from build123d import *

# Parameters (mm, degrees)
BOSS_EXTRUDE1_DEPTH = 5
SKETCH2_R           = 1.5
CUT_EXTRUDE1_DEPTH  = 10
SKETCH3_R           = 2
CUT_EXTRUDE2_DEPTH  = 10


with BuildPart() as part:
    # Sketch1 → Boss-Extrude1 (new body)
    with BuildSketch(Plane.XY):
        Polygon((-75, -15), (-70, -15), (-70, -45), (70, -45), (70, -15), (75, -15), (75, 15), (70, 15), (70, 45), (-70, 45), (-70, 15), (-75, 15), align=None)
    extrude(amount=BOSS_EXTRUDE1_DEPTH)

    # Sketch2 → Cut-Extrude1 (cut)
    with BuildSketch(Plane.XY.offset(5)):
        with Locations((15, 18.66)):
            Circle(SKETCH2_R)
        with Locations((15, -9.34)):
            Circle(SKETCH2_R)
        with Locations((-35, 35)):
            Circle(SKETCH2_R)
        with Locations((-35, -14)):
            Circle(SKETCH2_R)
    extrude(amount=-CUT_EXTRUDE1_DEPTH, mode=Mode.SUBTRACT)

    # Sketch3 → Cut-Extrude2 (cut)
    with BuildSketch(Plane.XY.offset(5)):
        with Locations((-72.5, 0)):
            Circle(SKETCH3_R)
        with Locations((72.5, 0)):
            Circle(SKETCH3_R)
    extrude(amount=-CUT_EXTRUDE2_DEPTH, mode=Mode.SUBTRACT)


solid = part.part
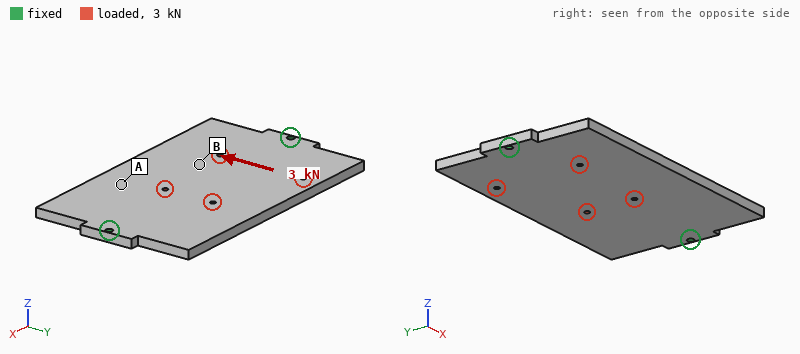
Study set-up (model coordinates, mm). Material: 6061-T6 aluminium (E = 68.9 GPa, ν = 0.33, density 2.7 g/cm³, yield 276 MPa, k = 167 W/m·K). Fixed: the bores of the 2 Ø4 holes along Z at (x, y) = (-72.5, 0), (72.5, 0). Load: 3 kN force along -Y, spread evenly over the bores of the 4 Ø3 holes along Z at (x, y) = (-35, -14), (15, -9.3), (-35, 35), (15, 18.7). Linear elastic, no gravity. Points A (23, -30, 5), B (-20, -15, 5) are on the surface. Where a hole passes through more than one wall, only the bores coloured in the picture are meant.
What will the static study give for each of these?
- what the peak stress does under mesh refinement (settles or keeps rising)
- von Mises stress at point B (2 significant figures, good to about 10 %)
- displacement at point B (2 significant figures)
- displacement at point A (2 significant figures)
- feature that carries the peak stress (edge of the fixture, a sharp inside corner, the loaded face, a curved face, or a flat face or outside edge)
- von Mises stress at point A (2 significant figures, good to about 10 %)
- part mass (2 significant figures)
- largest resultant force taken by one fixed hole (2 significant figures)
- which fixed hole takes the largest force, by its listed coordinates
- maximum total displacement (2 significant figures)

keeps rising
3.5 MPa
17 µm
15 µm
edge of the fixture
7.5 MPa
170 g
1.7 kN
(-72.5, 0)
18 µm
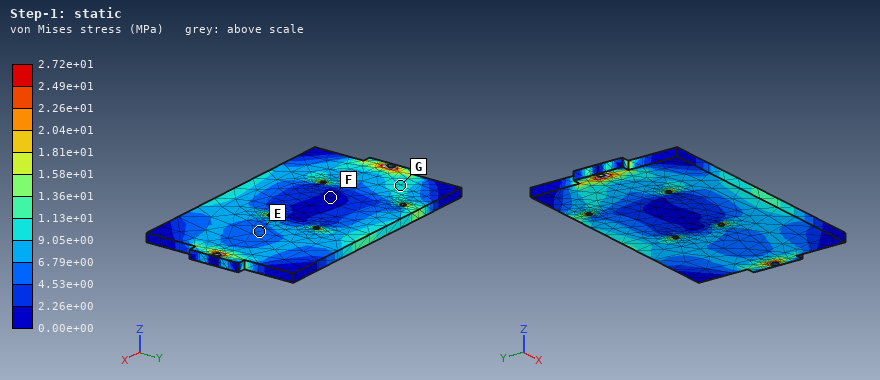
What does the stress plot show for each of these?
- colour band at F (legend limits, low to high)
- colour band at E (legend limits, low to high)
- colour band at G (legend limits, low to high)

0.00e+00 to 2.26e+00 MPa
4.53e+00 to 6.79e+00 MPa
9.05e+00 to 1.13e+01 MPa
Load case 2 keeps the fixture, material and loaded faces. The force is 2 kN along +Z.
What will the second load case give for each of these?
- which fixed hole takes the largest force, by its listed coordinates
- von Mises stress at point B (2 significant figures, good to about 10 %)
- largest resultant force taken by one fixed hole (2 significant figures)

(-72.5, 0)
51 MPa
1.2 kN
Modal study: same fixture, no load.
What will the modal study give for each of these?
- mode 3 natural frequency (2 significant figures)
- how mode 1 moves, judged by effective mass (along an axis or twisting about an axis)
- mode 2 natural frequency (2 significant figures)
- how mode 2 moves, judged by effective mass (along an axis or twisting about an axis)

1800 Hz
twisting about X
820 Hz
along Z
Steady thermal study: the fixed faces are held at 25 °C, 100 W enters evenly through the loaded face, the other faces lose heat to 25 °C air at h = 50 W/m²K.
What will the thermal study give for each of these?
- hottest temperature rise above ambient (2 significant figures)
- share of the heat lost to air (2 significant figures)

51 K
43 %
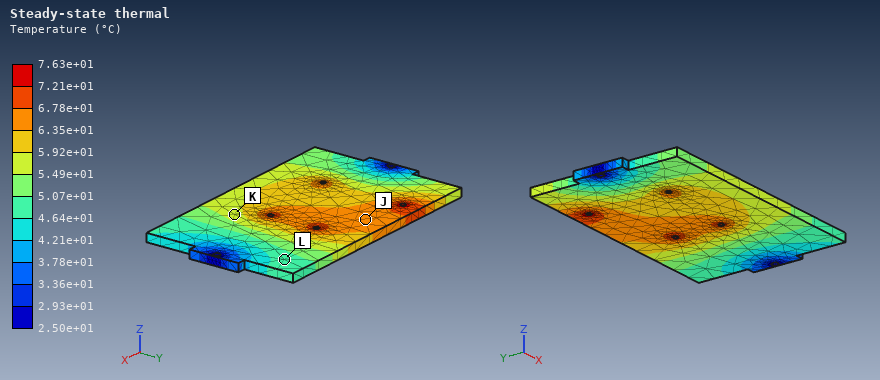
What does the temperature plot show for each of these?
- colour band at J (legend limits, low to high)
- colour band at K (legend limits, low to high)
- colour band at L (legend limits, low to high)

6.35e+01 to 6.78e+01 °C
5.49e+01 to 5.92e+01 °C
4.64e+01 to 5.07e+01 °C
